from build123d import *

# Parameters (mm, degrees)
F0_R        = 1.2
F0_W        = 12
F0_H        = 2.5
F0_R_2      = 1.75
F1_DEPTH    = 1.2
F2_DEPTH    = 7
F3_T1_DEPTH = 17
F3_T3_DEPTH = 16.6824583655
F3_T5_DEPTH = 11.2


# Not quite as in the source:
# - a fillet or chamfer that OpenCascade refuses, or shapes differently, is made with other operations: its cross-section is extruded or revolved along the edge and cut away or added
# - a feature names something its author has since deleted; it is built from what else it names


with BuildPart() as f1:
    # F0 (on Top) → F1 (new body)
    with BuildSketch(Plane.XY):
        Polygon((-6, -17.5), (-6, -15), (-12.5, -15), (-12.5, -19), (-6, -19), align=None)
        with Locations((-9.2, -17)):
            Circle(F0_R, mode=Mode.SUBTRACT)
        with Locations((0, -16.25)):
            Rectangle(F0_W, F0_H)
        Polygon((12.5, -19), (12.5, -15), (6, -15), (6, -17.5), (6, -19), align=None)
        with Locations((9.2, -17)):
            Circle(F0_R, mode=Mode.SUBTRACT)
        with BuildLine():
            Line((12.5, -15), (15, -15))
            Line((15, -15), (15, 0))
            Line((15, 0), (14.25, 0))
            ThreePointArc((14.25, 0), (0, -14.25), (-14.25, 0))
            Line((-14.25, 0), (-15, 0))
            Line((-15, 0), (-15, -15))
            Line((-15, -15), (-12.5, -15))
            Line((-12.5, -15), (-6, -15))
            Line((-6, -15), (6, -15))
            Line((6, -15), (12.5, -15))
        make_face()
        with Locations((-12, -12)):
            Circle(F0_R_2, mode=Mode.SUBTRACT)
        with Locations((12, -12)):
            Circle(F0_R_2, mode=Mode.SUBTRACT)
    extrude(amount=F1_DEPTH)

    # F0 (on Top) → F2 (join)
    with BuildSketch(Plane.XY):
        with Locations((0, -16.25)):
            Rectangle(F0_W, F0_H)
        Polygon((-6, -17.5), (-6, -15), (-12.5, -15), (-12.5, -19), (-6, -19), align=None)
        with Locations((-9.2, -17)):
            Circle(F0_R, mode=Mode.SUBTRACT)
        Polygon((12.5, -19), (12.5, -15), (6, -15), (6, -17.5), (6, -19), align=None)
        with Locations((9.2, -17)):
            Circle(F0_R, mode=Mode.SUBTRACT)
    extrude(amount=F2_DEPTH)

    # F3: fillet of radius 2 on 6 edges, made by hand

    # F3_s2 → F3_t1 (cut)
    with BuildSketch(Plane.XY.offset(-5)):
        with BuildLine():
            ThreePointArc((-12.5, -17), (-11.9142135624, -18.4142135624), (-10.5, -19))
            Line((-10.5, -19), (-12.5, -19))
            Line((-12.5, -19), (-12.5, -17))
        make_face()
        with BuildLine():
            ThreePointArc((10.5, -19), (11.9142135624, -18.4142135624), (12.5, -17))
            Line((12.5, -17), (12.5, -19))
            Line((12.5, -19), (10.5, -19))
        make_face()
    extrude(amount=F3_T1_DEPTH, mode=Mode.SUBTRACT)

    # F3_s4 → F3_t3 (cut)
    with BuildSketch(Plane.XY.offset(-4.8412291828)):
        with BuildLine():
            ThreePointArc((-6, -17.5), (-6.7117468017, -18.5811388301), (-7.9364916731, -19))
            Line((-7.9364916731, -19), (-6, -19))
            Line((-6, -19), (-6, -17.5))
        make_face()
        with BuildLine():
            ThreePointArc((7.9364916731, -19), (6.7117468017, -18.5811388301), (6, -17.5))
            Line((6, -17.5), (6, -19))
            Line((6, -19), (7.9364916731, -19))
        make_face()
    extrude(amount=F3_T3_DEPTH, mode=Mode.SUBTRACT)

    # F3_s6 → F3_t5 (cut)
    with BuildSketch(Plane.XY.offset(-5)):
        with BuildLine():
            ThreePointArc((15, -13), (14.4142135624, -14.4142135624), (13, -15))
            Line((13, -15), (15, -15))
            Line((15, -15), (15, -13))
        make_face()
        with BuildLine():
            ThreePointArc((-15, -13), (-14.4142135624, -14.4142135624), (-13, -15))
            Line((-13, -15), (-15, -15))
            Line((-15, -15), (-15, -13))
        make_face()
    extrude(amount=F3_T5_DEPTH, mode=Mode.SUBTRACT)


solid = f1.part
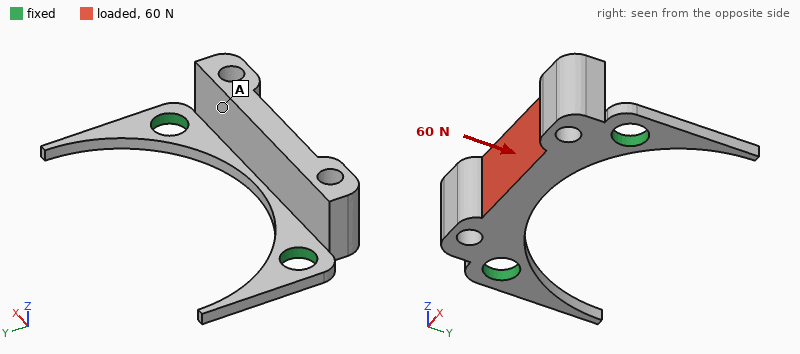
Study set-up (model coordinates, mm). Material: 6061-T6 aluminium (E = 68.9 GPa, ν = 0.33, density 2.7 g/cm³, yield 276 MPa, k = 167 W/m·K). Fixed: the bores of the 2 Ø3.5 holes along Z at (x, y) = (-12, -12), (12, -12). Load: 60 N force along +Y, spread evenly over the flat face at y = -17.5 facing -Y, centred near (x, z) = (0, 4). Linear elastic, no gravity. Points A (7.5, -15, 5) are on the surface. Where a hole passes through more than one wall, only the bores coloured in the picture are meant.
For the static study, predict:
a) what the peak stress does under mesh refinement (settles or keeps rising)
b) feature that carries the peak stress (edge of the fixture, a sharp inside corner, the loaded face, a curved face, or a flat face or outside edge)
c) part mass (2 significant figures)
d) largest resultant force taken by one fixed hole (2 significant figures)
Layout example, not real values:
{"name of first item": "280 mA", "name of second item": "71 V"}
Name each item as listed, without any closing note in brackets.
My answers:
{"what the peak stress does under mesh refinement": "keeps rising", "feature that carries the peak stress": "a sharp inside corner", "part mass": "1.7 g", "largest resultant force taken by one fixed hole": "41 N"}
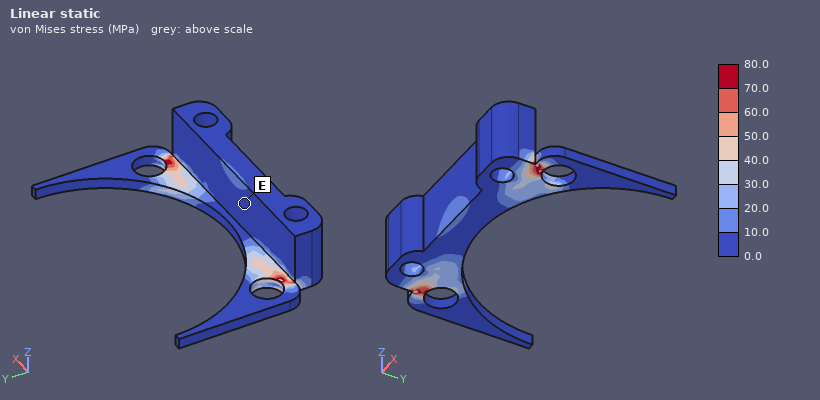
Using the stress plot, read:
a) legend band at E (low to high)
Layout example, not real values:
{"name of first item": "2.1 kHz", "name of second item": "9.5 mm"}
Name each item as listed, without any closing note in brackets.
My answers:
{"legend band at E": "0.0 to 10.0 MPa"}
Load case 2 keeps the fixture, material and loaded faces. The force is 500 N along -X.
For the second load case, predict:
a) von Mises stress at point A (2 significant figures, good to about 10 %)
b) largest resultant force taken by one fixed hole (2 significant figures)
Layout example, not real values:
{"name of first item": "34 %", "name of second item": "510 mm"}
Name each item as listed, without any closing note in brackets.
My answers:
{"von Mises stress at point A": "11 MPa", "largest resultant force taken by one fixed hole": "270 N"}
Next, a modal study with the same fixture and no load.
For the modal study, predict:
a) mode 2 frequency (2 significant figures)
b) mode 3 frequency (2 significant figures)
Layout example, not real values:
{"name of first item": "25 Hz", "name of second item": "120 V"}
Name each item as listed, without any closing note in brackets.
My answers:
{"mode 2 frequency": "15 kHz", "mode 3 frequency": "15 kHz"}
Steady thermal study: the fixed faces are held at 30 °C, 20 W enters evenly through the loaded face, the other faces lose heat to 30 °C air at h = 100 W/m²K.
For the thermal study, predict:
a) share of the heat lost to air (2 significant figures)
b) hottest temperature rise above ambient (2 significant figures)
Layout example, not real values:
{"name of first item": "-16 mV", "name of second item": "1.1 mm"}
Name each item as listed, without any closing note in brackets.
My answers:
{"share of the heat lost to air": "9.4 %", "hottest temperature rise above ambient": "45 K"}
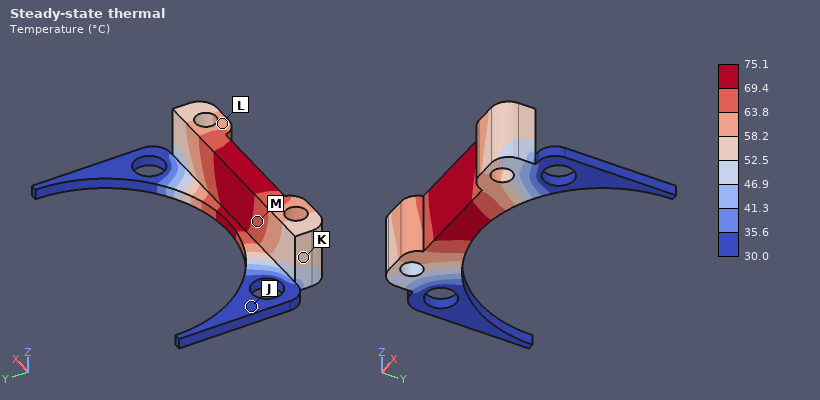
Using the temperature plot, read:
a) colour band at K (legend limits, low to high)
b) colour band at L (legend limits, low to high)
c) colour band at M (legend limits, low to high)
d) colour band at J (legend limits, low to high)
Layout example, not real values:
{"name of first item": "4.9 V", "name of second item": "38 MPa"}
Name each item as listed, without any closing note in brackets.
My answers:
{"colour band at K": "52.5 to 58.2 °C", "colour band at L": "58.2 to 63.8 °C", "colour band at M": "63.8 to 69.4 °C", "colour band at J": "30.0 to 35.6 °C"}
